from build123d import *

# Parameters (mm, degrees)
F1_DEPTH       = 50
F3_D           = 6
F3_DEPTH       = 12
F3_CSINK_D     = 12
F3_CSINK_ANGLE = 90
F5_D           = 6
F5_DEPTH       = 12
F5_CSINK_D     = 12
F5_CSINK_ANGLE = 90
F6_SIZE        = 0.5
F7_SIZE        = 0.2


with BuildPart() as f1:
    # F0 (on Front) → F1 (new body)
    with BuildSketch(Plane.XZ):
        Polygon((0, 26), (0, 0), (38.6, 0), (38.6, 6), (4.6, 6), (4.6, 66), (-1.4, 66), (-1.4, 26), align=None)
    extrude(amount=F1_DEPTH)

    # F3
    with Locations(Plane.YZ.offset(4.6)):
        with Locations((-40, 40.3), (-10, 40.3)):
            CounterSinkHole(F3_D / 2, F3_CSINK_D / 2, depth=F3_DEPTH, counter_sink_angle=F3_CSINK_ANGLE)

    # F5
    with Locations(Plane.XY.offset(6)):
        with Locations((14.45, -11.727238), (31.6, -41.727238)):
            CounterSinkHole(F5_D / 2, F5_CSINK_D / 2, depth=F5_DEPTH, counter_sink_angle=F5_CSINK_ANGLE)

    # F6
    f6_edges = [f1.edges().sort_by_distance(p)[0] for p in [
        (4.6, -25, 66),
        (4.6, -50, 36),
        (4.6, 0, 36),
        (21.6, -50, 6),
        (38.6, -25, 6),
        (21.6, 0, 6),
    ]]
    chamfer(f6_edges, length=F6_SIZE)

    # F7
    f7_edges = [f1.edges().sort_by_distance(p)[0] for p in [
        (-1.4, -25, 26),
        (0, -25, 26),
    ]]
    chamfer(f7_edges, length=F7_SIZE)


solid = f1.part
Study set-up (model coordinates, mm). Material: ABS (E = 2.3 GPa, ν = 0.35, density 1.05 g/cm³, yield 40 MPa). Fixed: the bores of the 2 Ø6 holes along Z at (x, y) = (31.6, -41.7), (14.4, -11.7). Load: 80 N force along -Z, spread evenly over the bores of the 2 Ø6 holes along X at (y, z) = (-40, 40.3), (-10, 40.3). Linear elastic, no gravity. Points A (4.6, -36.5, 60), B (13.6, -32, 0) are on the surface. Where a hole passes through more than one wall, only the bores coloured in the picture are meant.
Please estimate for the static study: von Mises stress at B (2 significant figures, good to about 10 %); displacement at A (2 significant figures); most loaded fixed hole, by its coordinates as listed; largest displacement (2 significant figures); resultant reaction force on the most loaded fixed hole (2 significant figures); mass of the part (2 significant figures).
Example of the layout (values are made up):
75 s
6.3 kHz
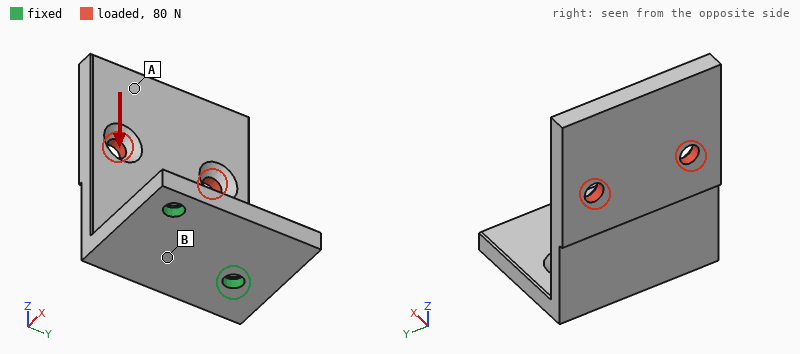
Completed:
2.3 MPa
0.88 mm
(14.4, -11.7)
1.0 mm
67 N
28 g
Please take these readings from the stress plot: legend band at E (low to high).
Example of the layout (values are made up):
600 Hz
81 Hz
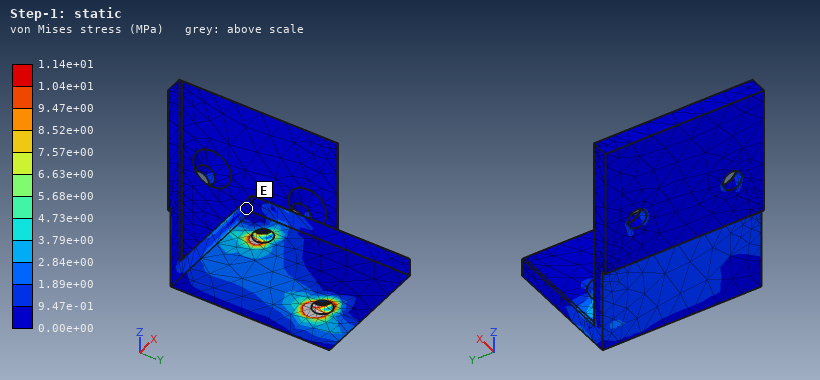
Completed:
0.00e+00 to 9.47e-01 MPa
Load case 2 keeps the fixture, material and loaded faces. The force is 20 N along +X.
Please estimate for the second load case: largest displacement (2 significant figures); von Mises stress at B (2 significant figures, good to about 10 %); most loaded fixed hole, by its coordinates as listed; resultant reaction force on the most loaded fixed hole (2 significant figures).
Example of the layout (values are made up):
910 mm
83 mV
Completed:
1.1 mm
1.7 MPa
(31.6, -41.7)
15 N
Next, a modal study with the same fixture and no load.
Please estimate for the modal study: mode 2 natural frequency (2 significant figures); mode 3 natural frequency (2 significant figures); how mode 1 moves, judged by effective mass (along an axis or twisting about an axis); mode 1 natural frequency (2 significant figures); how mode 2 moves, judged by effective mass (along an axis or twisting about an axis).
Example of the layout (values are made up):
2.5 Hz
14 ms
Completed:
430 Hz
810 Hz
along X
210 Hz
along Y
